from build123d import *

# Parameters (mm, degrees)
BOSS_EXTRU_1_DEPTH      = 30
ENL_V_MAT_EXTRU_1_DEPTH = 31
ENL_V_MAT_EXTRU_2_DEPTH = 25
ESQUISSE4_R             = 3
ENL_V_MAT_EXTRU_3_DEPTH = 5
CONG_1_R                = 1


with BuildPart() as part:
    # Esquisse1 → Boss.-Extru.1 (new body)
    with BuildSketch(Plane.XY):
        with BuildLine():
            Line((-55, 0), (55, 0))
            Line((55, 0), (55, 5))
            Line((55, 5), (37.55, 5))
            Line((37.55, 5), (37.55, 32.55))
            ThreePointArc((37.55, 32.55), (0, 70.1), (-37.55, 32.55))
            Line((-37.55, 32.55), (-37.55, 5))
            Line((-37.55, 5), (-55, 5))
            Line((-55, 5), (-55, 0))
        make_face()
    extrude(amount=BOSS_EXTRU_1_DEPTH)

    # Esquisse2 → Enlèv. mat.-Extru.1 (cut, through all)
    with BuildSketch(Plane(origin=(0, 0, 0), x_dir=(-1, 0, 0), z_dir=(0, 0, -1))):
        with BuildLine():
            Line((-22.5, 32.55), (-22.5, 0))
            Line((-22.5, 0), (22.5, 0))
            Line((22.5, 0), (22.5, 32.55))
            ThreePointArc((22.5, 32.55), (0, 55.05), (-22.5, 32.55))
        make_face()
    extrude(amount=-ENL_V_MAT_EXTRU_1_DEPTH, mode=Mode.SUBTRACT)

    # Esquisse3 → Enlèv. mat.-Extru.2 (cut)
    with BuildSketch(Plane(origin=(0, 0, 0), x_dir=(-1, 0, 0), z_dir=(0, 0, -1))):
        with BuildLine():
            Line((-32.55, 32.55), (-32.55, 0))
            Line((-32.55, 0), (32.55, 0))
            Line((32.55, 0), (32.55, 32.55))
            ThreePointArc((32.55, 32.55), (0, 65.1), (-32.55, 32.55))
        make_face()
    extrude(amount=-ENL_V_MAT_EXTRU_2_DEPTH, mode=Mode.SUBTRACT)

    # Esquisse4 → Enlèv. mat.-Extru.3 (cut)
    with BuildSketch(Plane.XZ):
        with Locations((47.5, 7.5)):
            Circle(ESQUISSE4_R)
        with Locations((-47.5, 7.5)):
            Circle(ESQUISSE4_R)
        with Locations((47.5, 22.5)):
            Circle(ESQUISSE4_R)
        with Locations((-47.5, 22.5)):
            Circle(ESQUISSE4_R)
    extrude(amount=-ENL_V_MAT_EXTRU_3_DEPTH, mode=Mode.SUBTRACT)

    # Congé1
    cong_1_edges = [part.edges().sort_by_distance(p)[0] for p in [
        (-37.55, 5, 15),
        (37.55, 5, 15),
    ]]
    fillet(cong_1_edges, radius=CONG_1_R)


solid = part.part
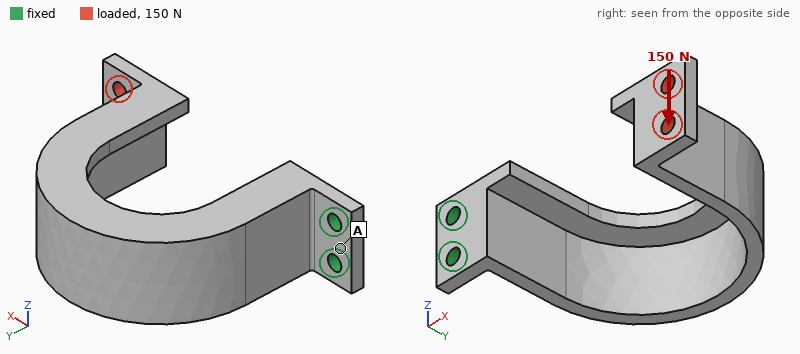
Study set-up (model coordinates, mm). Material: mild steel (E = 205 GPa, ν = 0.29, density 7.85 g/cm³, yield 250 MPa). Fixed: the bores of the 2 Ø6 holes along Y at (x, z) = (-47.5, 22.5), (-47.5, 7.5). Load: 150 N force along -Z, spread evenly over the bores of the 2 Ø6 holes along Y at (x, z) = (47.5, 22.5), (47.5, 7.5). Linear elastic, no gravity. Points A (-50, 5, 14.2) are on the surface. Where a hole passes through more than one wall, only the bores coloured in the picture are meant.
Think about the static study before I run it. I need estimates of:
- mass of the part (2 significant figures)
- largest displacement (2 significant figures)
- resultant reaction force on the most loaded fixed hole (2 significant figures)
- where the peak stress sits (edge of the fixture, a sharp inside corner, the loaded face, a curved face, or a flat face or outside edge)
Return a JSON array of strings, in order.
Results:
["300 g", "0.75 mm", "760 N", "a curved face"]
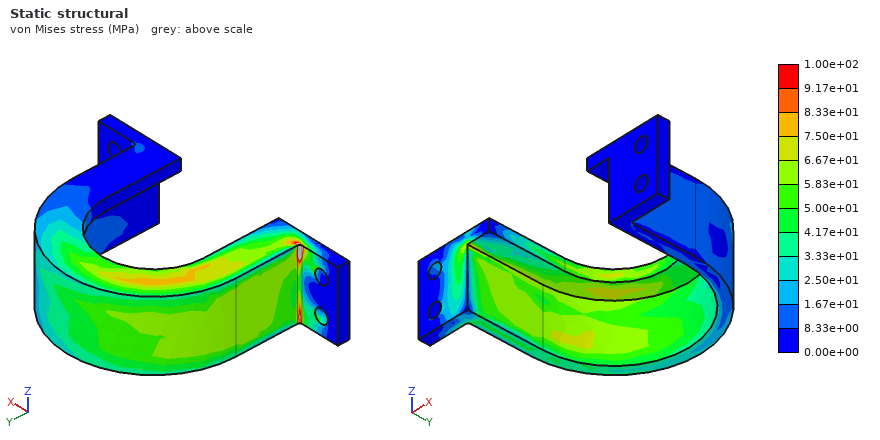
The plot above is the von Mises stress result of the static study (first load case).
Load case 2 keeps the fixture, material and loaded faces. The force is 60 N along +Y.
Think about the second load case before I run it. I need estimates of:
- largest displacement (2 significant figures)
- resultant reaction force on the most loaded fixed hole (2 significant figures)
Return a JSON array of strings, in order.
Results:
["0.20 mm", "49 N"]
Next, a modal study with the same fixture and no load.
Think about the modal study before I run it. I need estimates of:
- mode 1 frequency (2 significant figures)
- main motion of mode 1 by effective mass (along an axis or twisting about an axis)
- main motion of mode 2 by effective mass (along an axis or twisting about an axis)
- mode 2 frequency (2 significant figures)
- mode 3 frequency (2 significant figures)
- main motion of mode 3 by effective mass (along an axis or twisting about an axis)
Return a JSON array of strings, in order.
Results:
["260 Hz", "along Y", "along Z", "280 Hz", "700 Hz", "along X"]
